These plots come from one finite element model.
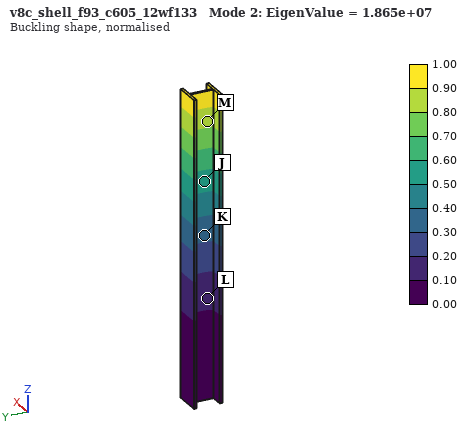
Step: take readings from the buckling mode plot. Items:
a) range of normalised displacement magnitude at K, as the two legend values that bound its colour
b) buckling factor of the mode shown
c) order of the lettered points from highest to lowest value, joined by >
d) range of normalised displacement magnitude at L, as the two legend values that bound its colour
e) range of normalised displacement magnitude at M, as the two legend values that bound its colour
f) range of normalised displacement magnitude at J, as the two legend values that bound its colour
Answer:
0.30 to 0.40
1.865e+07
M > J > K > L
0.10 to 0.20
0.80 to 0.90
0.50 to 0.60
